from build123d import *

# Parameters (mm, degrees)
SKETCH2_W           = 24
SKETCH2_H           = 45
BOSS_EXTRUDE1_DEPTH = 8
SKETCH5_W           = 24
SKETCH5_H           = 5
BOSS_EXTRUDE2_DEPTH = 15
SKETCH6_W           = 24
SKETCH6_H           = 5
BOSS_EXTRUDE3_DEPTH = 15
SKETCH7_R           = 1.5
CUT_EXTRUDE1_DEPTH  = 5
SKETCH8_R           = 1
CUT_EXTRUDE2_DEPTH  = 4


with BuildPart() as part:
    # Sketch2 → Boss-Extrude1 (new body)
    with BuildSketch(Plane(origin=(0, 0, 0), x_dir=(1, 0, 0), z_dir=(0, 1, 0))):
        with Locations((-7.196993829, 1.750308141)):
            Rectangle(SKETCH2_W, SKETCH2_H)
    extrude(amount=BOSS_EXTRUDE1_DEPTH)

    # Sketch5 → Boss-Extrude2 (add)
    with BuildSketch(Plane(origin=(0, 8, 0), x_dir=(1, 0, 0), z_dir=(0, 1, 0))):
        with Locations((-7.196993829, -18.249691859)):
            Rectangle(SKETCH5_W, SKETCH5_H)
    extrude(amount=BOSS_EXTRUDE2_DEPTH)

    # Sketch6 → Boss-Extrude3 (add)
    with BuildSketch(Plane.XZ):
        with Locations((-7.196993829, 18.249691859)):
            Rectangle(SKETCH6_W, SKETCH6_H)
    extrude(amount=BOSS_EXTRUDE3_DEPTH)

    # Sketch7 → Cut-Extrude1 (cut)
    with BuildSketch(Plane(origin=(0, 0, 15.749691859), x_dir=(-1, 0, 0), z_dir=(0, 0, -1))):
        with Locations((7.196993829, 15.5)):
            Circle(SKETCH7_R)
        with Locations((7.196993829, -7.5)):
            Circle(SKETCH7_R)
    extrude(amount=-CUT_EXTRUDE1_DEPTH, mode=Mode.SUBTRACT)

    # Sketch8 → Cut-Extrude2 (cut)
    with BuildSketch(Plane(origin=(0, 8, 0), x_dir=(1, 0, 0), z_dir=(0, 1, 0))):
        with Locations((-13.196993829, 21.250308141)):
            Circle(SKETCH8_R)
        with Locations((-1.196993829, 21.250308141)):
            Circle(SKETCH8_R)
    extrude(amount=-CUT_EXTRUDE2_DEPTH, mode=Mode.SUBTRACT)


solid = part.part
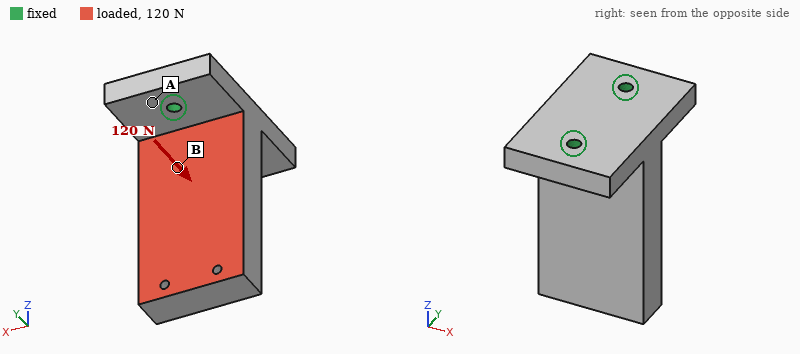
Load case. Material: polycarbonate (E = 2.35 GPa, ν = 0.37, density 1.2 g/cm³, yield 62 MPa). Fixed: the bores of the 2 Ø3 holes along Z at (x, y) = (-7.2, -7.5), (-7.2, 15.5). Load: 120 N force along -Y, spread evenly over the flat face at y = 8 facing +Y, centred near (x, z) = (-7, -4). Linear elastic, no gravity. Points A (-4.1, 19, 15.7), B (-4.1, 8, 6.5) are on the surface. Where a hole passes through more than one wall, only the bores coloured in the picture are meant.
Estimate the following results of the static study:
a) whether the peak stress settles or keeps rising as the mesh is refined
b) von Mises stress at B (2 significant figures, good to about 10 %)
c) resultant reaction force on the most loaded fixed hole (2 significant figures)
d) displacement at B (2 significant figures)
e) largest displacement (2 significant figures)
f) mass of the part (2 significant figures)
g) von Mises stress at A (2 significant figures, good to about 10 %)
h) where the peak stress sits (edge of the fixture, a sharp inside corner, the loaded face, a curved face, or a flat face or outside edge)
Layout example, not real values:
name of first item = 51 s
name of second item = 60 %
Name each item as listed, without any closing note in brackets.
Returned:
whether the peak stress settles or keeps rising as the mesh is refined = keeps rising
von Mises stress at B = 5.3 MPa
resultant reaction force on the most loaded fixed hole = 150 N
displacement at B = 0.13 mm
largest displacement = 0.67 mm
mass of the part = 15 g
von Mises stress at A = 2.0 MPa
where the peak stress sits = edge of the fixture
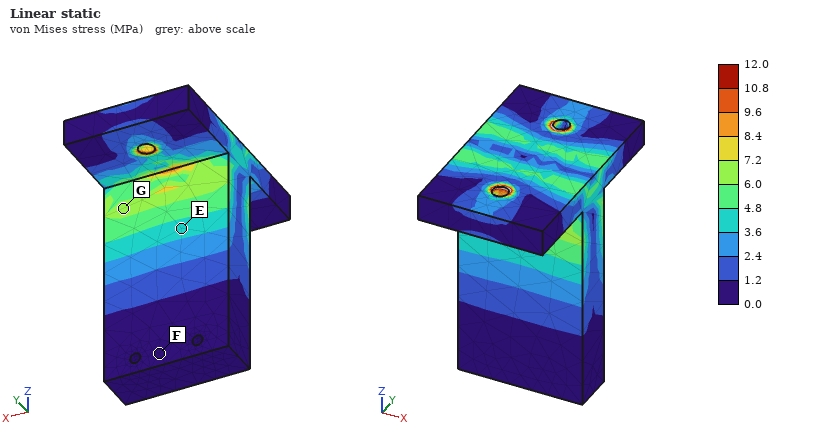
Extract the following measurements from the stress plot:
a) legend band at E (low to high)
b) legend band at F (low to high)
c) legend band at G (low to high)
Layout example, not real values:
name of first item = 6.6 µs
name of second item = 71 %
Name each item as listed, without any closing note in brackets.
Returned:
legend band at E = 3.6 to 4.8 MPa
legend band at F = 0.0 to 1.2 MPa
legend band at G = 6.0 to 7.2 MPa
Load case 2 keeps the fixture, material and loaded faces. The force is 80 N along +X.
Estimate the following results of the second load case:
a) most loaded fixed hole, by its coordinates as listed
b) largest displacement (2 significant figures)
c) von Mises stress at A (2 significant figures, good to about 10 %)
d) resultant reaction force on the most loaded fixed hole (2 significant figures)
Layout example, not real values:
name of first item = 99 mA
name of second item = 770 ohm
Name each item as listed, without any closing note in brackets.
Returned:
most loaded fixed hole, by its coordinates as listed = (-7.2, 15.5)
largest displacement = 0.51 mm
von Mises stress at A = 3.4 MPa
resultant reaction force on the most loaded fixed hole = 53 N
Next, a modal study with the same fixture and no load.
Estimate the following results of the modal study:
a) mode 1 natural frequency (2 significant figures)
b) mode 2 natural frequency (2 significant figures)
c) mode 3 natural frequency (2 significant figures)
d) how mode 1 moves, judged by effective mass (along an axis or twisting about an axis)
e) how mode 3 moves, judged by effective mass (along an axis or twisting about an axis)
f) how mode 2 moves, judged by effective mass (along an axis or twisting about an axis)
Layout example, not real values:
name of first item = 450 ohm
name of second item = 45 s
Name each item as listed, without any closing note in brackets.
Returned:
mode 1 natural frequency = 790 Hz
mode 2 natural frequency = 870 Hz
mode 3 natural frequency = 3000 Hz
how mode 1 moves, judged by effective mass = along X
how mode 3 moves, judged by effective mass = twisting about Z
how mode 2 moves, judged by effective mass = along Y
